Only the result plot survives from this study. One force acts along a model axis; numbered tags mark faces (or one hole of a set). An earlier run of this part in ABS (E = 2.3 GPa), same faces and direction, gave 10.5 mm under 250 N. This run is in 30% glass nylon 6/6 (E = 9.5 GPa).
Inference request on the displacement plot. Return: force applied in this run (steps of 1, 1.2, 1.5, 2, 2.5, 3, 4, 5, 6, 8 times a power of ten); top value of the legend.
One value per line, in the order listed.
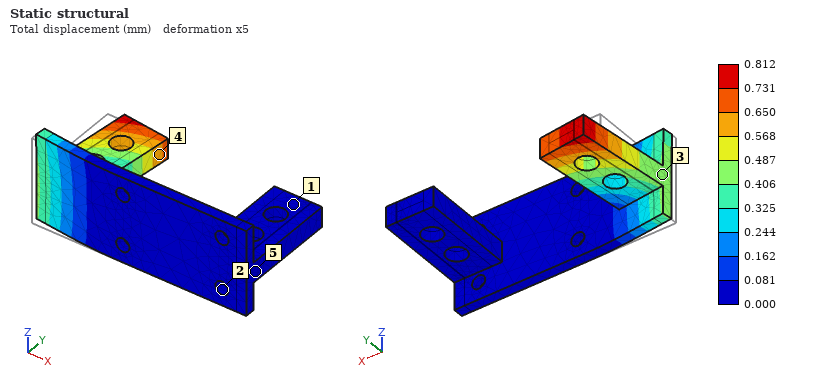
80 N
0.812 mm
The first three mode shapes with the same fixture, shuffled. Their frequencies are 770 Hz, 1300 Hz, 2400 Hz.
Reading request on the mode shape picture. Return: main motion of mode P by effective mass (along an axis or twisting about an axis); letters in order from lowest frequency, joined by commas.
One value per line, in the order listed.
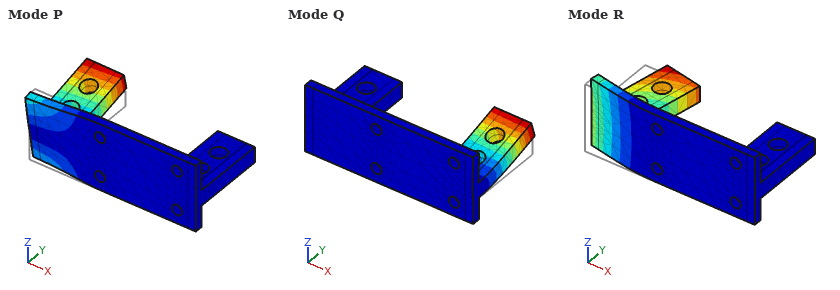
along Z
R, P, Q
